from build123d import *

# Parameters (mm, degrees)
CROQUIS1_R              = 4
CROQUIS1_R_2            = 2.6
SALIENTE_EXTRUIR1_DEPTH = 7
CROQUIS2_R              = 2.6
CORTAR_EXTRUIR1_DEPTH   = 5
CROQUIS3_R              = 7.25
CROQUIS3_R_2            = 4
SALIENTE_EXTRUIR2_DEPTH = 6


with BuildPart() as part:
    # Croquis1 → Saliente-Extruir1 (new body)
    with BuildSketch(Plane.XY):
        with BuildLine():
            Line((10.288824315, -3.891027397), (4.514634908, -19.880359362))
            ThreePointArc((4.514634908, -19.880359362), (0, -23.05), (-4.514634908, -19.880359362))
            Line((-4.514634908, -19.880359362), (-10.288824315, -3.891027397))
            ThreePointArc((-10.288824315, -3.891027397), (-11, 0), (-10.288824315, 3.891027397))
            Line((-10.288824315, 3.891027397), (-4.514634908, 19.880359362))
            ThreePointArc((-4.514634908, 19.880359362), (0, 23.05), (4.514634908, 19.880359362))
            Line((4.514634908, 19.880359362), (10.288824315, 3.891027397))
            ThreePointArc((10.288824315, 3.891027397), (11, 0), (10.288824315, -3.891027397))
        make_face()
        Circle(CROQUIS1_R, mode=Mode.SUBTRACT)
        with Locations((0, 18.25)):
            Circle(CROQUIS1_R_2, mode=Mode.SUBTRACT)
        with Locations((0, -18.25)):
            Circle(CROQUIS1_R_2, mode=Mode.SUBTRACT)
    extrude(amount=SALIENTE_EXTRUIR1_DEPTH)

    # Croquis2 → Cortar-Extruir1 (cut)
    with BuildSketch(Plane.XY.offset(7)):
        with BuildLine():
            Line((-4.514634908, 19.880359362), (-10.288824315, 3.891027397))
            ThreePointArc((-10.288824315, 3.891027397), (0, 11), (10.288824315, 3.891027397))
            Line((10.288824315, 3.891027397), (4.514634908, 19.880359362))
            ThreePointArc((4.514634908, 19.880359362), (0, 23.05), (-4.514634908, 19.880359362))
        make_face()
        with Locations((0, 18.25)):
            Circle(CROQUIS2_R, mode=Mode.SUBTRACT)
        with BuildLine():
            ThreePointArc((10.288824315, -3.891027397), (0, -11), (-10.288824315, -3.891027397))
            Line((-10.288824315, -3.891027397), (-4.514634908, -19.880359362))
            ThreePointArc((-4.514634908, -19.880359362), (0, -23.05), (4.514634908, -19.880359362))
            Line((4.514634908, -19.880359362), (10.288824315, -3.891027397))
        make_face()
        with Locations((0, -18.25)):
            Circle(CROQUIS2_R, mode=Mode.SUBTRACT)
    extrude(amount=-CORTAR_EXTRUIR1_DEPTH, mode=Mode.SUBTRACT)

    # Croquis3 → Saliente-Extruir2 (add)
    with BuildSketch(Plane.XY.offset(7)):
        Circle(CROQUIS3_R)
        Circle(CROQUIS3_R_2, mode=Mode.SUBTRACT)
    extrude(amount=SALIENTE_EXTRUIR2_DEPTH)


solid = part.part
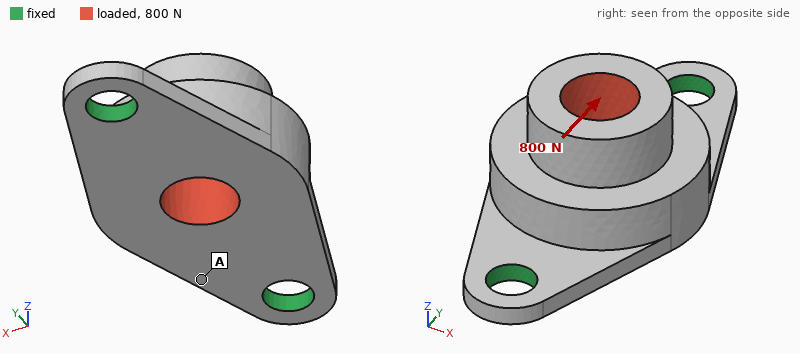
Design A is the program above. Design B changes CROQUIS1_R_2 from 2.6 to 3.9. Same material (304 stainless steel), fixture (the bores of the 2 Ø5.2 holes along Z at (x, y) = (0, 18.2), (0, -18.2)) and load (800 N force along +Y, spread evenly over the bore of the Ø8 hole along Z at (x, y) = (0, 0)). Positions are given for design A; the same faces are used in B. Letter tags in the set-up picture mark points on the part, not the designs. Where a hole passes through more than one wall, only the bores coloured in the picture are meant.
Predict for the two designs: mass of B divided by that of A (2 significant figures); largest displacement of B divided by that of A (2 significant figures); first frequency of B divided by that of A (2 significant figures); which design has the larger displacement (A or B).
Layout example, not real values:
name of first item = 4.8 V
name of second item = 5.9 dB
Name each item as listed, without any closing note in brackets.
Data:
mass of B divided by that of A = 0.97
largest displacement of B divided by that of A = 0.66
first frequency of B divided by that of A = 1.3
which design has the larger displacement = A
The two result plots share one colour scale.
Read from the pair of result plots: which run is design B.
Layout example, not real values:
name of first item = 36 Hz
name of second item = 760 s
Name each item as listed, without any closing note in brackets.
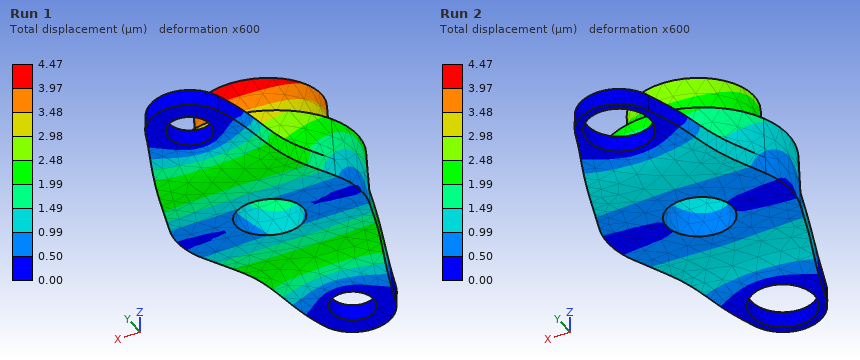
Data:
which run is design B = Run 2
